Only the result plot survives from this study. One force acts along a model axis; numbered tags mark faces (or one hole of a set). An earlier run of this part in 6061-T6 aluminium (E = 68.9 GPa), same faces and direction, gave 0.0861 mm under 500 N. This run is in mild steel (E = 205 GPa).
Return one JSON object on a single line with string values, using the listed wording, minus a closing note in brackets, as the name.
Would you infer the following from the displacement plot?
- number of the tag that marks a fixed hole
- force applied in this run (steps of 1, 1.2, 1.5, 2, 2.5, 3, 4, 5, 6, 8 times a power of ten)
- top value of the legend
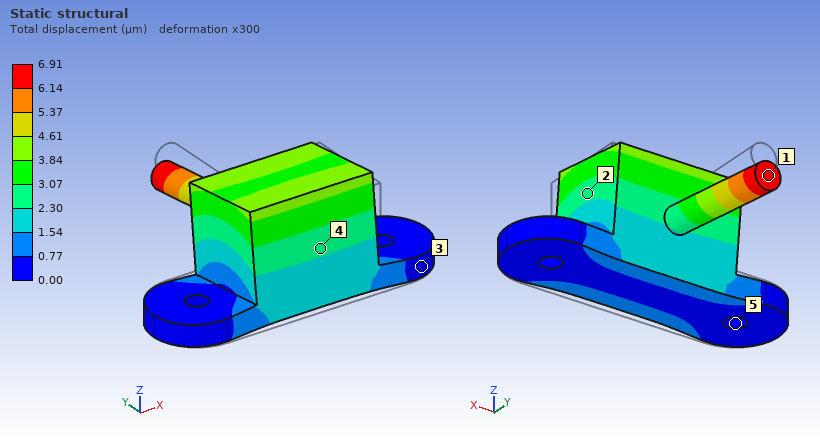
{"number of the tag that marks a fixed hole": "5", "force applied in this run": "120 N", "top value of the legend": "6.91 µm"}
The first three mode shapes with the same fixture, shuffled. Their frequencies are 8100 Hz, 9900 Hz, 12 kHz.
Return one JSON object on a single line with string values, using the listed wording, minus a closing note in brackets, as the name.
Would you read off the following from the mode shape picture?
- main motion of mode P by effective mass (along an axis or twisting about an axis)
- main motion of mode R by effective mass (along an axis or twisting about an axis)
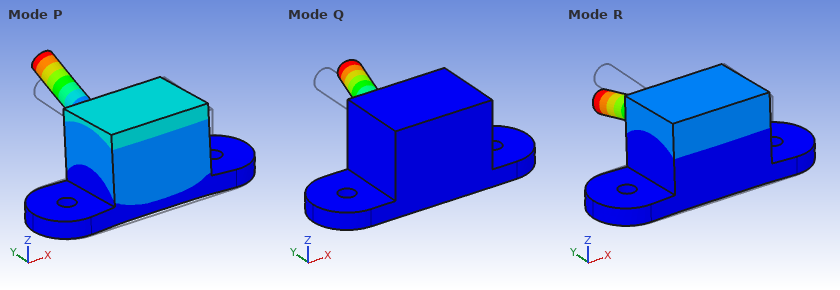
{"main motion of mode P by effective mass": "along Y", "main motion of mode R by effective mass": "along Y"}
